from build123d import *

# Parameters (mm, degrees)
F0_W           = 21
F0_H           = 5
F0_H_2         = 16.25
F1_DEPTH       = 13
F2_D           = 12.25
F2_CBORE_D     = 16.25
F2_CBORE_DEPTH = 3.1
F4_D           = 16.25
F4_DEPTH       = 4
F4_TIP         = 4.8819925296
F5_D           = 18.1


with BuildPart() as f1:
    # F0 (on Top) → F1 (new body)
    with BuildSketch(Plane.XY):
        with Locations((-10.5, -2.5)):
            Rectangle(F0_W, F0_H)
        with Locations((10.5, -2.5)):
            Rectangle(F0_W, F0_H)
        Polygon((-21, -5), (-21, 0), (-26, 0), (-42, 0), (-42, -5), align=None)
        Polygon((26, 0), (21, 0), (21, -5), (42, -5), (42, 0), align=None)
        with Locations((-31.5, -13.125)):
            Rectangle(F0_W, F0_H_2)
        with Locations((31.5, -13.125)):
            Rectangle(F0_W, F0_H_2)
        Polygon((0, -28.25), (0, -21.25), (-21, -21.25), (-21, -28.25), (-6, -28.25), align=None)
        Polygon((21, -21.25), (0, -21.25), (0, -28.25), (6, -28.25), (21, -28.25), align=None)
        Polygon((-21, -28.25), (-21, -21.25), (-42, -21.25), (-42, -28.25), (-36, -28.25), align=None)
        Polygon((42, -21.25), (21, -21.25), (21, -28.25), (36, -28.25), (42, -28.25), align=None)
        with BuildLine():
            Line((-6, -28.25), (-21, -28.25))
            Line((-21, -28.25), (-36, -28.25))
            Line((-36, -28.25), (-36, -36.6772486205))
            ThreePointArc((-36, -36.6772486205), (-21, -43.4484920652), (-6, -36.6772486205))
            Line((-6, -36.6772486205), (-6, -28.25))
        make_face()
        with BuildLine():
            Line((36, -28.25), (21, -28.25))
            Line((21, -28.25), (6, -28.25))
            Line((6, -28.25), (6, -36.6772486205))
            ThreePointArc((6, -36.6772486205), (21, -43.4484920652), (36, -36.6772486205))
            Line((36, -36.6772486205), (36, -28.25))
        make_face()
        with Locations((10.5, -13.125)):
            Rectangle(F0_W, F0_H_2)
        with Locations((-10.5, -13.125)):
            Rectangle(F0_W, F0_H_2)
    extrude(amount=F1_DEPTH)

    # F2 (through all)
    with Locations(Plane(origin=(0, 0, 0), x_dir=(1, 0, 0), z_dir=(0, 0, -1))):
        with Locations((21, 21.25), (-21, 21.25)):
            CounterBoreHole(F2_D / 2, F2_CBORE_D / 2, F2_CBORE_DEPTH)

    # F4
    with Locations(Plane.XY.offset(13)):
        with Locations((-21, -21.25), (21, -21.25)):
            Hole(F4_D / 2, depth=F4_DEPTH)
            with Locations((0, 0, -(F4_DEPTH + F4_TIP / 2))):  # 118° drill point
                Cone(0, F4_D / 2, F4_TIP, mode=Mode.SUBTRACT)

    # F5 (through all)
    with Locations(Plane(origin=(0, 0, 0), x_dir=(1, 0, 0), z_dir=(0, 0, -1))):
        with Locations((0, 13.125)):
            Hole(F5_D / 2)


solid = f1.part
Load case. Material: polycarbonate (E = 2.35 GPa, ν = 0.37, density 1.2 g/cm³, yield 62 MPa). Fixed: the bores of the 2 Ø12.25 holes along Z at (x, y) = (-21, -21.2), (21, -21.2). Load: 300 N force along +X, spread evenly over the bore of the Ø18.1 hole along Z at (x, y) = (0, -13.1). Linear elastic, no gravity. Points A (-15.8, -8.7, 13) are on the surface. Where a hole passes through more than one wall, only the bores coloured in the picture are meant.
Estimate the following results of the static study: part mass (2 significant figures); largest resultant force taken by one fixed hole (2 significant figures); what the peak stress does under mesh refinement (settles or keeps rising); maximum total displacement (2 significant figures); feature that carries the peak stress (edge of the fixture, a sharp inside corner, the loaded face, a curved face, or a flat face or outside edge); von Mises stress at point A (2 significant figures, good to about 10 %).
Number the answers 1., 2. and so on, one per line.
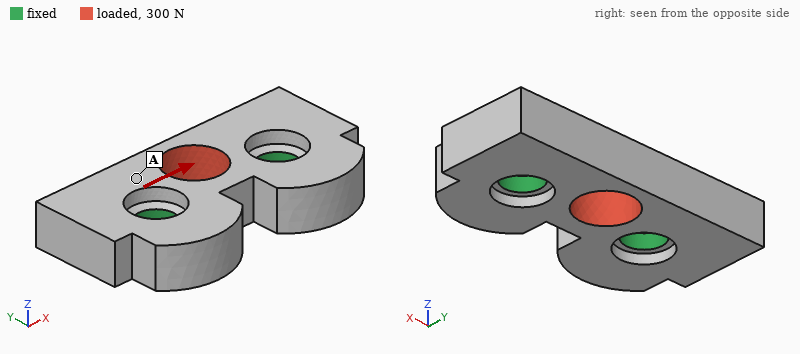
1. 40 g
2. 150 N
3. keeps rising
4. 12 µm
5. edge of the fixture
6. 0.52 MPa
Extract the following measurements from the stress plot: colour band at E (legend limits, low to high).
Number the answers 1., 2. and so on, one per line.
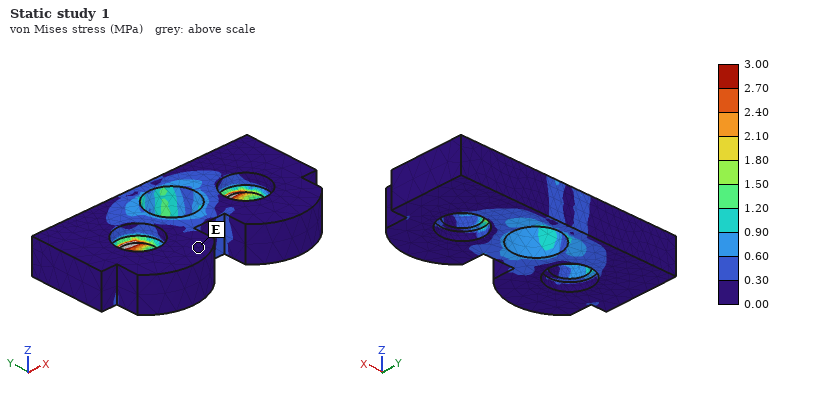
1. 0.00 to 0.30 MPa
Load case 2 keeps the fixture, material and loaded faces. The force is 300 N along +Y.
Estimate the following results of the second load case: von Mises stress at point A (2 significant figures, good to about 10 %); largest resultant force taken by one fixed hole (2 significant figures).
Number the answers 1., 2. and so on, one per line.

1. 0.51 MPa
2. 160 N
